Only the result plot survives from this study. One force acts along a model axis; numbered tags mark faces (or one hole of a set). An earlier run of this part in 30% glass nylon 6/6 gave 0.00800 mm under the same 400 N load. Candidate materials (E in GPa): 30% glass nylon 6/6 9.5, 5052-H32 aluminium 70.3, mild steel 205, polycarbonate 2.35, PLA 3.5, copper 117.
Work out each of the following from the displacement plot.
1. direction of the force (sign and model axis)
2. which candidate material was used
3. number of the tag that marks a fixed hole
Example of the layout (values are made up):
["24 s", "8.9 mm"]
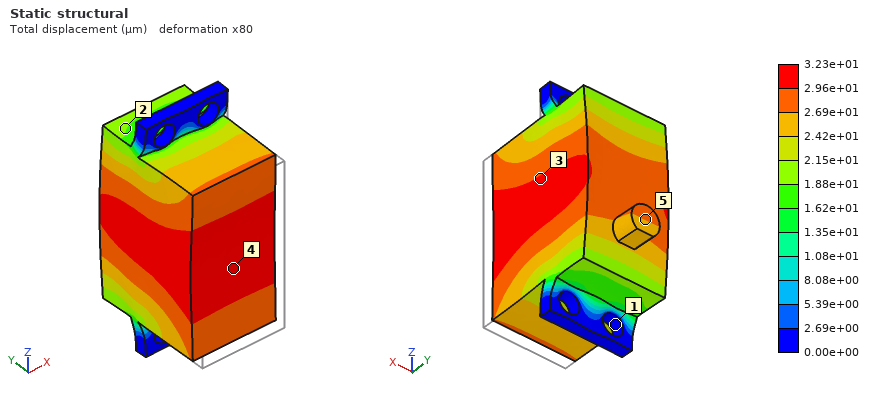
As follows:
["+Y", "polycarbonate", "1"]
